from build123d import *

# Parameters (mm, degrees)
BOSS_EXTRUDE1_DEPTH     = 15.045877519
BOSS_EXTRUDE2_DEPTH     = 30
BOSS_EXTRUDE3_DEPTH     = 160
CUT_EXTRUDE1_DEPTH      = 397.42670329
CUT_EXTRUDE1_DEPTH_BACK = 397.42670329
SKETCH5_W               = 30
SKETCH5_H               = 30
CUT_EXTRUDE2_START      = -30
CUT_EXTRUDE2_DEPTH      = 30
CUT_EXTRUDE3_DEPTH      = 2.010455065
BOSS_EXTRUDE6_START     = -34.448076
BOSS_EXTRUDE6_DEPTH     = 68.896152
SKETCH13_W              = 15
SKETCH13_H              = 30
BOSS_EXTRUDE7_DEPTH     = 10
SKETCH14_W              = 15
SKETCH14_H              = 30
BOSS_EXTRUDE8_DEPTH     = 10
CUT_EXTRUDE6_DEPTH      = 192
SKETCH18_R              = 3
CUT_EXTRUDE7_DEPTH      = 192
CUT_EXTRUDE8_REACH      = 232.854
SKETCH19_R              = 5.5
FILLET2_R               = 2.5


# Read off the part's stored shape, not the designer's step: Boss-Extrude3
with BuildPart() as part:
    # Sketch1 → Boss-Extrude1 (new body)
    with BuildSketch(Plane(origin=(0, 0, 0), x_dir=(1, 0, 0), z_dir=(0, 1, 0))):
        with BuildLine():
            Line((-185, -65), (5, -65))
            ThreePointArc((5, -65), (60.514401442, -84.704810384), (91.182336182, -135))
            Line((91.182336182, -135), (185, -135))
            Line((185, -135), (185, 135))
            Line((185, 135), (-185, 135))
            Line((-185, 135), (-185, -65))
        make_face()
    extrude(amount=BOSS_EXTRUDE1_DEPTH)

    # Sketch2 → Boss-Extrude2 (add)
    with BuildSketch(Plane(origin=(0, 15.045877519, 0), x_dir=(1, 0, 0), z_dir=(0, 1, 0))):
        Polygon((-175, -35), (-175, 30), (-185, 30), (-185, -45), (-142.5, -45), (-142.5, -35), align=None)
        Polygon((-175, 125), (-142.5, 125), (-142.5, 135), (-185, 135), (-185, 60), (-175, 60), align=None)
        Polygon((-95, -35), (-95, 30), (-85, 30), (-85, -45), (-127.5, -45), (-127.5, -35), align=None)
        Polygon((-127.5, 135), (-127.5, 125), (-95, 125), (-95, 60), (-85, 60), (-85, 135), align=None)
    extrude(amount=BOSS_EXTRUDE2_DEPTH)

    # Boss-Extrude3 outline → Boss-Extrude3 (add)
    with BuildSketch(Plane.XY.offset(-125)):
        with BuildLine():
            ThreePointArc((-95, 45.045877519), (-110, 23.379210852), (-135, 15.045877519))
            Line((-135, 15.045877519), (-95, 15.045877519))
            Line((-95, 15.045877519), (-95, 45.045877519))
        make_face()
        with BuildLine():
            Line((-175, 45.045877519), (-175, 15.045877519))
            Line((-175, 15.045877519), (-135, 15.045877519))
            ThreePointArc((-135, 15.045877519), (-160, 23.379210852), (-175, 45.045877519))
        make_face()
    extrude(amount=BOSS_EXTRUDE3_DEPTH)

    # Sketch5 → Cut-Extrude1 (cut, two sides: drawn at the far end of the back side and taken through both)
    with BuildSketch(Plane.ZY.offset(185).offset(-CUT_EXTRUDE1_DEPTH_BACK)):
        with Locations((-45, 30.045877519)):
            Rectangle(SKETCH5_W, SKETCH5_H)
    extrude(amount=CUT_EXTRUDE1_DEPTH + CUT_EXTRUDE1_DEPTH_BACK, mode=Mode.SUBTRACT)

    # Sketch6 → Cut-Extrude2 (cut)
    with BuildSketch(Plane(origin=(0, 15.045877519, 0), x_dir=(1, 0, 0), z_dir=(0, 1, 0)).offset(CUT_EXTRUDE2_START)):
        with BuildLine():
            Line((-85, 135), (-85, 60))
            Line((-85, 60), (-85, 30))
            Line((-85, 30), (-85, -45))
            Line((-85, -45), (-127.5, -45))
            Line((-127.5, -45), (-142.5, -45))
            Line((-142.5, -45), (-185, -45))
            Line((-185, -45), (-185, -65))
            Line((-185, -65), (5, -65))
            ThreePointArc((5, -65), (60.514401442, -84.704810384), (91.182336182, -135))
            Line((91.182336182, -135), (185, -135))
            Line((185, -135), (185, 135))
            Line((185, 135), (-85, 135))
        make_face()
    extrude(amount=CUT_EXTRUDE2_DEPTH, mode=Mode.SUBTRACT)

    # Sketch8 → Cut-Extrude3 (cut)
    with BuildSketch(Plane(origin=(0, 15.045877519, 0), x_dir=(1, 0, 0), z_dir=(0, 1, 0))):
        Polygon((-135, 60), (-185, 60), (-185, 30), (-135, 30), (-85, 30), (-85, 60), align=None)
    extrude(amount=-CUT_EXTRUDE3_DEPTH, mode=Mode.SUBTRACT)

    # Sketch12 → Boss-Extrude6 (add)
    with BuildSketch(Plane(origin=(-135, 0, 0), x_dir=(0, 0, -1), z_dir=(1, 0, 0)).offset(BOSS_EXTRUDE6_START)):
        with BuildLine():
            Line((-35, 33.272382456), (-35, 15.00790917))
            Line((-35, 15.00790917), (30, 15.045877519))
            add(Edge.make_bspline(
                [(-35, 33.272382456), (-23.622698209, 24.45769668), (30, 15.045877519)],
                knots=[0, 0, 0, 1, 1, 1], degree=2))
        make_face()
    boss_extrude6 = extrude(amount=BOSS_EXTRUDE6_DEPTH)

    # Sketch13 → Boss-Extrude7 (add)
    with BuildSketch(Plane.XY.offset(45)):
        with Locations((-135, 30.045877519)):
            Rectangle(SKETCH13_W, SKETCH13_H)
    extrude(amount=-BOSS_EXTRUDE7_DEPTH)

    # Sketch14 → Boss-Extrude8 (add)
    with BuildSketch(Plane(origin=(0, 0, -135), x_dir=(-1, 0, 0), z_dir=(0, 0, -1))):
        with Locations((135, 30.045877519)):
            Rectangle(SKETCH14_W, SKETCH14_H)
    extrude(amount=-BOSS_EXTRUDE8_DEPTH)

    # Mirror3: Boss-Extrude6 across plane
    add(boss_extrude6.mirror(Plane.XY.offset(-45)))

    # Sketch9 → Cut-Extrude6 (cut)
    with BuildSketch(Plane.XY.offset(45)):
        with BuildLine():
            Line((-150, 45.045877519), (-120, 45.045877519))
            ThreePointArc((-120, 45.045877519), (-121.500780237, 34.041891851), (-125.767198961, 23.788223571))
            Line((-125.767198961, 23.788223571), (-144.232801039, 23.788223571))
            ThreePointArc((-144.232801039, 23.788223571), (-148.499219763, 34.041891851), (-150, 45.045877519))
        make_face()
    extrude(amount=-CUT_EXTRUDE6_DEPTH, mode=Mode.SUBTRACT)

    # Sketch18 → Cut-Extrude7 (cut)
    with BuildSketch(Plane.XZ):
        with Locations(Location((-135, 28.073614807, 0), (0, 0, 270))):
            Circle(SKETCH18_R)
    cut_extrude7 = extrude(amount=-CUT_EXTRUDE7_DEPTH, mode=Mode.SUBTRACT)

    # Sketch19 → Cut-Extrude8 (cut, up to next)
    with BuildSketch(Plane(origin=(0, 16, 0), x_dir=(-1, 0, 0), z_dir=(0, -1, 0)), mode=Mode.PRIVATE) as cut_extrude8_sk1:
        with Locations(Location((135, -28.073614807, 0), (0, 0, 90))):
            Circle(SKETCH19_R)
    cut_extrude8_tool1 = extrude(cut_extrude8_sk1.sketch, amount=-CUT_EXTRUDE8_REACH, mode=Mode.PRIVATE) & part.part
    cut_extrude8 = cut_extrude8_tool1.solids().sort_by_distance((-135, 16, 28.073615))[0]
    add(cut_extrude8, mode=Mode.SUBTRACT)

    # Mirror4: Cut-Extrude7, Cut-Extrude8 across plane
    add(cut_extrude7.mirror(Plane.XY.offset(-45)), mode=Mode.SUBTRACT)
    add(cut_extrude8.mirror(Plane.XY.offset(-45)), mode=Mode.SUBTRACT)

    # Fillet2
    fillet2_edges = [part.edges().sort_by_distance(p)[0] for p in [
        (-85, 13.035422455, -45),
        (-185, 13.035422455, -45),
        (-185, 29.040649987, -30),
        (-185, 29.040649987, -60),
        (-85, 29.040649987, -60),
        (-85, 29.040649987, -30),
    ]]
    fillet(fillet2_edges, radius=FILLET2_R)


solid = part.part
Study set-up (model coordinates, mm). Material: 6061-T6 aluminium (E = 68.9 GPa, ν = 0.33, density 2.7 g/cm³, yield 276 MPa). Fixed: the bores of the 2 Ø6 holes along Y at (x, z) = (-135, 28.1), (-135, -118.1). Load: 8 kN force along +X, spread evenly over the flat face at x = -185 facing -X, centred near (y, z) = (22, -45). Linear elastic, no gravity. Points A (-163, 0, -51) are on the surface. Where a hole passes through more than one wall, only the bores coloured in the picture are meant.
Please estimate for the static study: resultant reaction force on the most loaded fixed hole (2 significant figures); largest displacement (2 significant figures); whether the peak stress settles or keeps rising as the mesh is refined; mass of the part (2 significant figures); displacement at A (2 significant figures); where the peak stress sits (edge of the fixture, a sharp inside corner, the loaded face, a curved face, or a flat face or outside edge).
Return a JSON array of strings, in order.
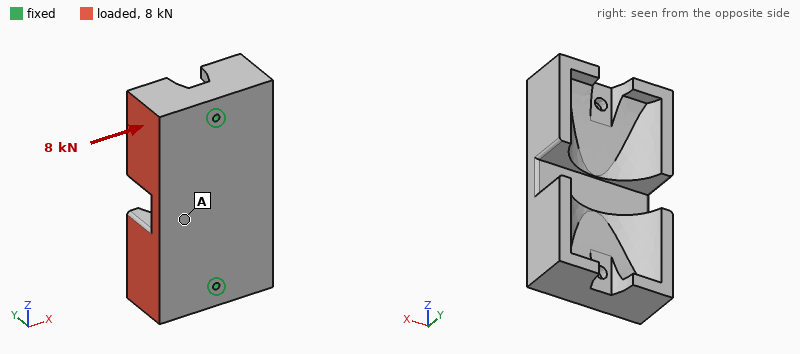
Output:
["4.0 kN", "50 µm", "keeps rising", "1.4 kg", "17 µm", "edge of the fixture"]
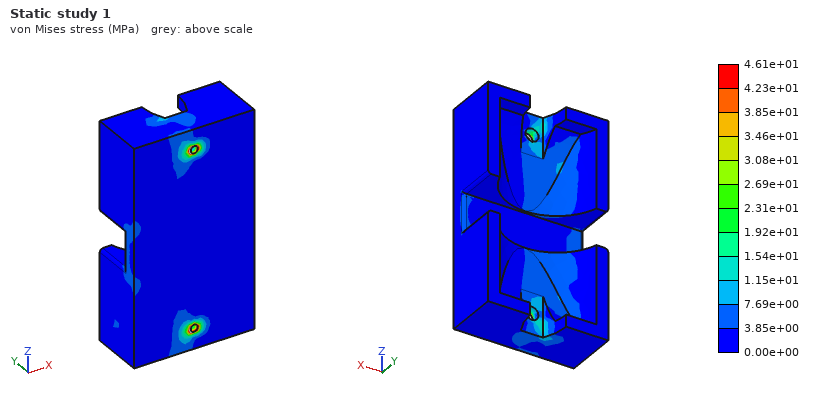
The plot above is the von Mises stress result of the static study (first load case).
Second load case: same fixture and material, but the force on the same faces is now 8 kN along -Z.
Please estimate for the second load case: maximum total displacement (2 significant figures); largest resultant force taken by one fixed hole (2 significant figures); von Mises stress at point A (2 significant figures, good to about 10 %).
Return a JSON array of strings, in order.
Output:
["15 µm", "4.9 kN", "4.1 MPa"]
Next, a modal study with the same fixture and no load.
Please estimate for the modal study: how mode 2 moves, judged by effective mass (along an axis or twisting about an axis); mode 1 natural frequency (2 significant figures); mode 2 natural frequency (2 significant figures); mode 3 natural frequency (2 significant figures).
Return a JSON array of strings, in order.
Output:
["along Y", "1700 Hz", "2000 Hz", "2900 Hz"]
